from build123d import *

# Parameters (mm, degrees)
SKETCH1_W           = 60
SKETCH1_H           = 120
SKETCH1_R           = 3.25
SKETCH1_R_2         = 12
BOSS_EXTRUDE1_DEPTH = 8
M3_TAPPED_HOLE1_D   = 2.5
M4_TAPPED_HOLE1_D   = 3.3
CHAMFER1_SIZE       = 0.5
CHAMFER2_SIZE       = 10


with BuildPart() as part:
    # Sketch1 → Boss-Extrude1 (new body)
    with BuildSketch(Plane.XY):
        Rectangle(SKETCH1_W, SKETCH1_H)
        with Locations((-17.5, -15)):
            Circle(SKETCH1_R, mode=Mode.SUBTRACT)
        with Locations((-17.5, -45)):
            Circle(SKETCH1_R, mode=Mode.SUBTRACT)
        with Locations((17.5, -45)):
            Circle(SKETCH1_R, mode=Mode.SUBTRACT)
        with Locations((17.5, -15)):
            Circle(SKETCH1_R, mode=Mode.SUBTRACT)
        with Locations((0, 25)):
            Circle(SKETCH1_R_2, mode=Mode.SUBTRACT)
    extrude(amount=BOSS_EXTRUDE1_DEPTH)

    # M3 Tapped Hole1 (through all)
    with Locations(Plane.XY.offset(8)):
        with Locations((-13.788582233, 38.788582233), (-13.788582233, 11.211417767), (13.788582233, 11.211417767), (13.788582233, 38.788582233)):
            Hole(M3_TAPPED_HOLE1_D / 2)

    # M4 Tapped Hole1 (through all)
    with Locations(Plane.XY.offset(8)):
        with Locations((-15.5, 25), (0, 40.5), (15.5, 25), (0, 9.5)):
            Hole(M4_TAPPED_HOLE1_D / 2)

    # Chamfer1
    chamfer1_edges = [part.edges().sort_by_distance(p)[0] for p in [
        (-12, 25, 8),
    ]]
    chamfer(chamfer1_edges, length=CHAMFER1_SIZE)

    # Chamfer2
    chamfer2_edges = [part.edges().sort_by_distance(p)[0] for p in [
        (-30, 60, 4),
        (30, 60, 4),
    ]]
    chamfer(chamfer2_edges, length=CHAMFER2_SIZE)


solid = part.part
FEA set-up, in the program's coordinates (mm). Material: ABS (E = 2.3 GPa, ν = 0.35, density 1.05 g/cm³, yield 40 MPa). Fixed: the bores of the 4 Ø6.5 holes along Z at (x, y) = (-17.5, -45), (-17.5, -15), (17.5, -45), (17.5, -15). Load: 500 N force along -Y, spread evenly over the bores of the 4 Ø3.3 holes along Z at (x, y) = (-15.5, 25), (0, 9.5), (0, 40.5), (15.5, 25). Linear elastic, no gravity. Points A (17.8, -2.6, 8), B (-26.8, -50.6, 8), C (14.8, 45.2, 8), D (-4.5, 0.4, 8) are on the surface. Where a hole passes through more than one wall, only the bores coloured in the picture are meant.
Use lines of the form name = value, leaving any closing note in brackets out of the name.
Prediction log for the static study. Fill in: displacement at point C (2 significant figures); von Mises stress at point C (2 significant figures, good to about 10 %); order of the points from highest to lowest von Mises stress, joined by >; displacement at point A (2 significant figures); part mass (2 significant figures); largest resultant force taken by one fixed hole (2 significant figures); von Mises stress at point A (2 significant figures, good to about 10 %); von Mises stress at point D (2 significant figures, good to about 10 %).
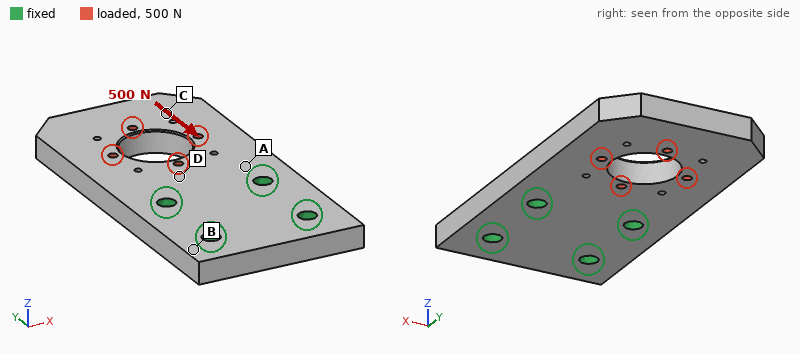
displacement at point C = 29 µm
von Mises stress at point C = 0.58 MPa
order of the points from highest to lowest von Mises stress, joined by > = A > D > C > B
displacement at point A = 6.9 µm
part mass = 54 g
largest resultant force taken by one fixed hole = 210 N
von Mises stress at point A = 1.3 MPa
von Mises stress at point D = 0.94 MPa
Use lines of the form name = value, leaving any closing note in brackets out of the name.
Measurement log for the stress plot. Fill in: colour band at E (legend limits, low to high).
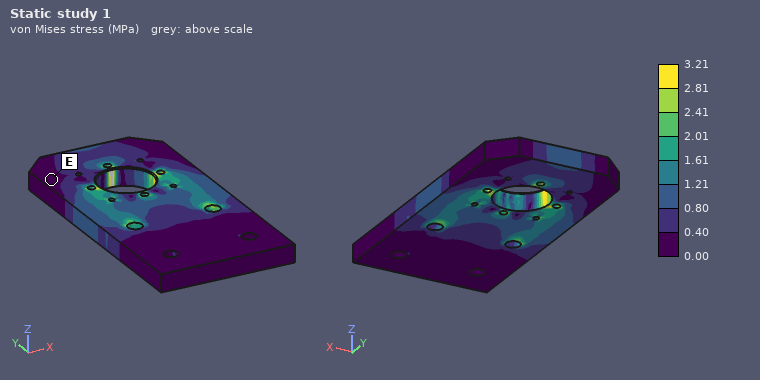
colour band at E = 0.00 to 0.40 MPa
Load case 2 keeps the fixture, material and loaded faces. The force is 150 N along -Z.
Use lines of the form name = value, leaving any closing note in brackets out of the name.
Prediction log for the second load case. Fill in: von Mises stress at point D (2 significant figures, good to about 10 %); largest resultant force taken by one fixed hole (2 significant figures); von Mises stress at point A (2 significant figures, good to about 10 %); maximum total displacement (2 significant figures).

von Mises stress at point D = 4.7 MPa
largest resultant force taken by one fixed hole = 100 N
von Mises stress at point A = 6.5 MPa
maximum total displacement = 1.4 mm
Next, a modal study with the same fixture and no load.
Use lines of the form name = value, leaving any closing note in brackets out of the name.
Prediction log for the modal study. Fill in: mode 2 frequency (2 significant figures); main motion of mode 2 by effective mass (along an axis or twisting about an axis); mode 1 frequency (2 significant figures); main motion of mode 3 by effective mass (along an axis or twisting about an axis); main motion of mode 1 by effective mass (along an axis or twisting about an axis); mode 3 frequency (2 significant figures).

mode 2 frequency = 910 Hz
main motion of mode 2 by effective mass = twisting about Y
mode 1 frequency = 350 Hz
main motion of mode 3 by effective mass = along X
main motion of mode 1 by effective mass = along Z
mode 3 frequency = 1600 Hz
